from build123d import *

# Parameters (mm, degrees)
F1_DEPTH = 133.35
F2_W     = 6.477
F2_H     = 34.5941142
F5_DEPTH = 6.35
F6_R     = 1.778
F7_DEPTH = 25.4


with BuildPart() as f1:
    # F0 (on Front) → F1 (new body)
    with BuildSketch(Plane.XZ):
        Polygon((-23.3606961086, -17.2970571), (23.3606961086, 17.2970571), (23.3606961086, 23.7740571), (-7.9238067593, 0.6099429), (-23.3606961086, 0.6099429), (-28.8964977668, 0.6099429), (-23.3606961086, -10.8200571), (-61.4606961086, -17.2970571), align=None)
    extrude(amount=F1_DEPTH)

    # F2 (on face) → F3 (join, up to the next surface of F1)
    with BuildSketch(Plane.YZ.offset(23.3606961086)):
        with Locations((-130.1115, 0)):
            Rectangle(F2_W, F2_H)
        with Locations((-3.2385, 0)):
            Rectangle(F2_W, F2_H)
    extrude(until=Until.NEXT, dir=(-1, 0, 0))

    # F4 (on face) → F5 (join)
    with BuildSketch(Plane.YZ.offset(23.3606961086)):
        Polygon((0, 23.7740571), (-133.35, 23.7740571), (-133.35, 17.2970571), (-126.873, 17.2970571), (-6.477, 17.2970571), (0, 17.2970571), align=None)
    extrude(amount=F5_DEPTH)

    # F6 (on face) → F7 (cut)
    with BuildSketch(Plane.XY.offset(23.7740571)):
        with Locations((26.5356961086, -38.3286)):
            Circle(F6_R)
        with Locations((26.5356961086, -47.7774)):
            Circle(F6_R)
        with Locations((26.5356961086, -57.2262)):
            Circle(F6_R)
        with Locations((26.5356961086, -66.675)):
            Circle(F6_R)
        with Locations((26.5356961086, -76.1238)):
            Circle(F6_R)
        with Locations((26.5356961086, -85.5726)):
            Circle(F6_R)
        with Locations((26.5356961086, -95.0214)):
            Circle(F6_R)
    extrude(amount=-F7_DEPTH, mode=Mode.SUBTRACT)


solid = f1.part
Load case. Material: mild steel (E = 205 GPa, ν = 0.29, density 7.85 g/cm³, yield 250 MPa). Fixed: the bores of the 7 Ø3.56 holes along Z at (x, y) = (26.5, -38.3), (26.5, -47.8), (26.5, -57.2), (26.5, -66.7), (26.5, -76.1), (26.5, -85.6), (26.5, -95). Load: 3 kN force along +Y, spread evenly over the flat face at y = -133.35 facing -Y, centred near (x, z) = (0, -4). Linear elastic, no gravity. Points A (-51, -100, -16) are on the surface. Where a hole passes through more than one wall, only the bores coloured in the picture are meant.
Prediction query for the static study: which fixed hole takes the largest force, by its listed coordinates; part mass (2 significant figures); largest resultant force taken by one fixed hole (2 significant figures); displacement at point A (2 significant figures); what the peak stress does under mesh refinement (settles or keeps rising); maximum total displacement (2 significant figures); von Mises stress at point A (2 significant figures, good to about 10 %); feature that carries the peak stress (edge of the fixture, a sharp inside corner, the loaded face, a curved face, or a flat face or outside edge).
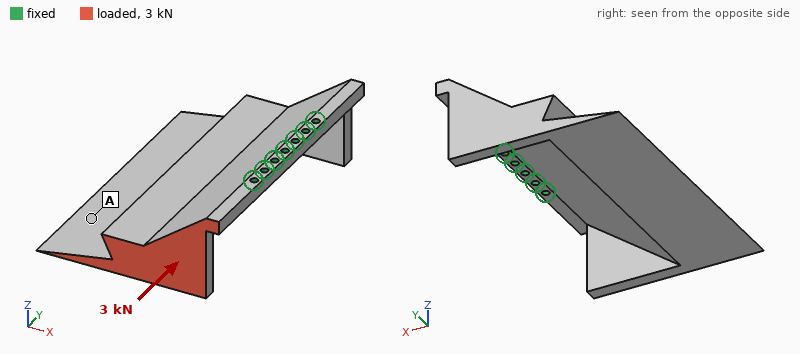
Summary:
(26.5, -95)
690 g
1.6 kN
0.031 mm
keeps rising
0.11 mm
9.0 MPa
edge of the fixture
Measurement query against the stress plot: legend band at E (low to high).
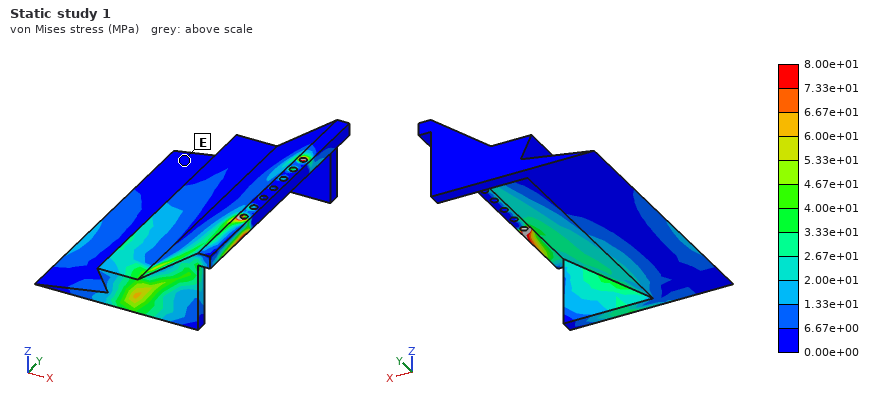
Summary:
0.00e+00 to 6.67e+00 MPa
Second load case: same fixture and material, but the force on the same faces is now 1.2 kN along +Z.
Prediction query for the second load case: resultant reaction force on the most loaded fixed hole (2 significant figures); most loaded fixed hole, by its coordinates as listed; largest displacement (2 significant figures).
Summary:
1.5 kN
(26.5, -95)
0.35 mm
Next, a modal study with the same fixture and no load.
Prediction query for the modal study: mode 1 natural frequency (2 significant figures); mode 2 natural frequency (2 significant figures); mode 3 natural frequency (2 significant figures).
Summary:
530 Hz
860 Hz
2400 Hz
